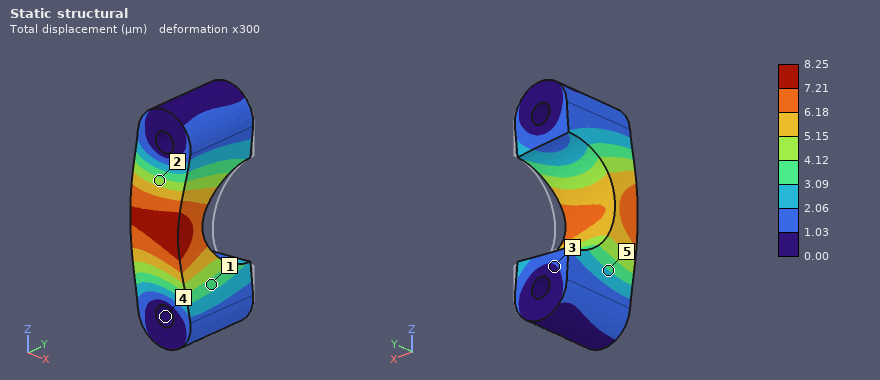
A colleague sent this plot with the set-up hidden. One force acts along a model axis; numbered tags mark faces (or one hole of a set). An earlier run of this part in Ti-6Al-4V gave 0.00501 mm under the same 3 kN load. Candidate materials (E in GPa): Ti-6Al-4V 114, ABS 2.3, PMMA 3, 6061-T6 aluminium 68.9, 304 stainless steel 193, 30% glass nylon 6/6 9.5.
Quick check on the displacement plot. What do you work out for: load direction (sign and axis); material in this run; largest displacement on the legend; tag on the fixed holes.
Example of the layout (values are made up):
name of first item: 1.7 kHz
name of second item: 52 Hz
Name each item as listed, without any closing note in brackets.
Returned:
load direction: -X
material in this run: 6061-T6 aluminium
largest displacement on the legend: 8.25 µm
tag on the fixed holes: 4
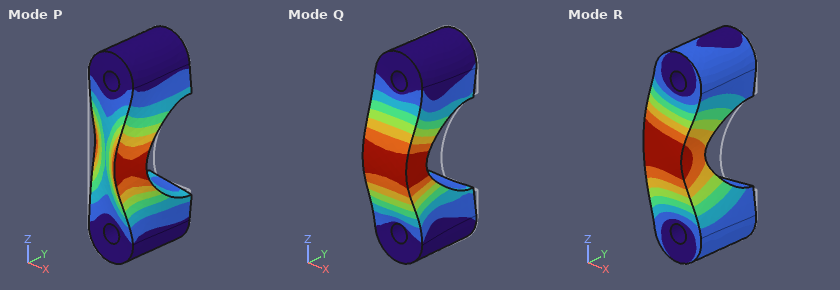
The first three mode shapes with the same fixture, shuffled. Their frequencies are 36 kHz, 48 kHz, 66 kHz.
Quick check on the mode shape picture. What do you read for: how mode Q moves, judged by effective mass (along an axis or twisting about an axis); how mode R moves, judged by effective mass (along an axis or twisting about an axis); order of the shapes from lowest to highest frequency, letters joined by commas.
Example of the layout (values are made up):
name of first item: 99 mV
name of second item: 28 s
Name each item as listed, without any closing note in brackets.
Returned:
how mode Q moves, judged by effective mass: along Y
how mode R moves, judged by effective mass: along X
order of the shapes from lowest to highest frequency, letters joined by commas: R, Q, P
